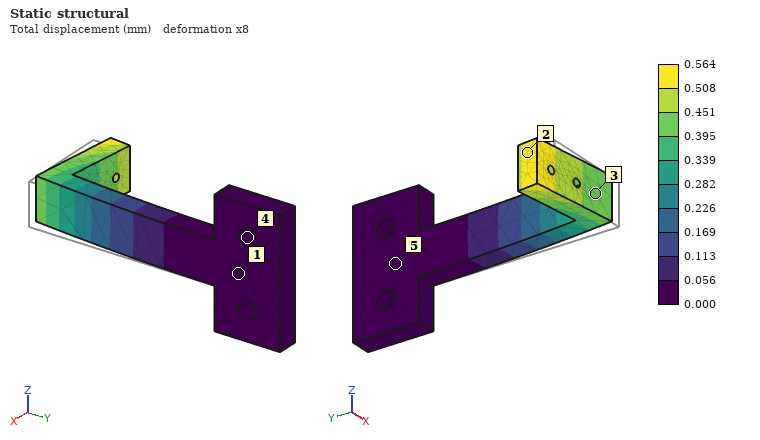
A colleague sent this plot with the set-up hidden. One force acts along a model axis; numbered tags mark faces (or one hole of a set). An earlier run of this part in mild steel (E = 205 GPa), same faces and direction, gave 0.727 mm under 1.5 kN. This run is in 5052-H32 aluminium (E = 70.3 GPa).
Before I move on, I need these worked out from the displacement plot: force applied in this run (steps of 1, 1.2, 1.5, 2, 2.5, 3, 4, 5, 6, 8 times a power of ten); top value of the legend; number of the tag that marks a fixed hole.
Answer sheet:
400 N
0.564 mm
4
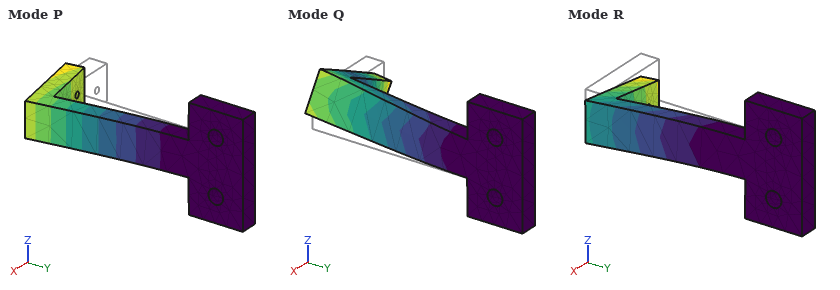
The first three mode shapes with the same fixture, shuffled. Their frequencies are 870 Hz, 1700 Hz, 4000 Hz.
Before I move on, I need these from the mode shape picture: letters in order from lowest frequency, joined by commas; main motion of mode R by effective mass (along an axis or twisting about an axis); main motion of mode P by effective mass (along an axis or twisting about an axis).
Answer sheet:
P, R, Q
along Z
along X
